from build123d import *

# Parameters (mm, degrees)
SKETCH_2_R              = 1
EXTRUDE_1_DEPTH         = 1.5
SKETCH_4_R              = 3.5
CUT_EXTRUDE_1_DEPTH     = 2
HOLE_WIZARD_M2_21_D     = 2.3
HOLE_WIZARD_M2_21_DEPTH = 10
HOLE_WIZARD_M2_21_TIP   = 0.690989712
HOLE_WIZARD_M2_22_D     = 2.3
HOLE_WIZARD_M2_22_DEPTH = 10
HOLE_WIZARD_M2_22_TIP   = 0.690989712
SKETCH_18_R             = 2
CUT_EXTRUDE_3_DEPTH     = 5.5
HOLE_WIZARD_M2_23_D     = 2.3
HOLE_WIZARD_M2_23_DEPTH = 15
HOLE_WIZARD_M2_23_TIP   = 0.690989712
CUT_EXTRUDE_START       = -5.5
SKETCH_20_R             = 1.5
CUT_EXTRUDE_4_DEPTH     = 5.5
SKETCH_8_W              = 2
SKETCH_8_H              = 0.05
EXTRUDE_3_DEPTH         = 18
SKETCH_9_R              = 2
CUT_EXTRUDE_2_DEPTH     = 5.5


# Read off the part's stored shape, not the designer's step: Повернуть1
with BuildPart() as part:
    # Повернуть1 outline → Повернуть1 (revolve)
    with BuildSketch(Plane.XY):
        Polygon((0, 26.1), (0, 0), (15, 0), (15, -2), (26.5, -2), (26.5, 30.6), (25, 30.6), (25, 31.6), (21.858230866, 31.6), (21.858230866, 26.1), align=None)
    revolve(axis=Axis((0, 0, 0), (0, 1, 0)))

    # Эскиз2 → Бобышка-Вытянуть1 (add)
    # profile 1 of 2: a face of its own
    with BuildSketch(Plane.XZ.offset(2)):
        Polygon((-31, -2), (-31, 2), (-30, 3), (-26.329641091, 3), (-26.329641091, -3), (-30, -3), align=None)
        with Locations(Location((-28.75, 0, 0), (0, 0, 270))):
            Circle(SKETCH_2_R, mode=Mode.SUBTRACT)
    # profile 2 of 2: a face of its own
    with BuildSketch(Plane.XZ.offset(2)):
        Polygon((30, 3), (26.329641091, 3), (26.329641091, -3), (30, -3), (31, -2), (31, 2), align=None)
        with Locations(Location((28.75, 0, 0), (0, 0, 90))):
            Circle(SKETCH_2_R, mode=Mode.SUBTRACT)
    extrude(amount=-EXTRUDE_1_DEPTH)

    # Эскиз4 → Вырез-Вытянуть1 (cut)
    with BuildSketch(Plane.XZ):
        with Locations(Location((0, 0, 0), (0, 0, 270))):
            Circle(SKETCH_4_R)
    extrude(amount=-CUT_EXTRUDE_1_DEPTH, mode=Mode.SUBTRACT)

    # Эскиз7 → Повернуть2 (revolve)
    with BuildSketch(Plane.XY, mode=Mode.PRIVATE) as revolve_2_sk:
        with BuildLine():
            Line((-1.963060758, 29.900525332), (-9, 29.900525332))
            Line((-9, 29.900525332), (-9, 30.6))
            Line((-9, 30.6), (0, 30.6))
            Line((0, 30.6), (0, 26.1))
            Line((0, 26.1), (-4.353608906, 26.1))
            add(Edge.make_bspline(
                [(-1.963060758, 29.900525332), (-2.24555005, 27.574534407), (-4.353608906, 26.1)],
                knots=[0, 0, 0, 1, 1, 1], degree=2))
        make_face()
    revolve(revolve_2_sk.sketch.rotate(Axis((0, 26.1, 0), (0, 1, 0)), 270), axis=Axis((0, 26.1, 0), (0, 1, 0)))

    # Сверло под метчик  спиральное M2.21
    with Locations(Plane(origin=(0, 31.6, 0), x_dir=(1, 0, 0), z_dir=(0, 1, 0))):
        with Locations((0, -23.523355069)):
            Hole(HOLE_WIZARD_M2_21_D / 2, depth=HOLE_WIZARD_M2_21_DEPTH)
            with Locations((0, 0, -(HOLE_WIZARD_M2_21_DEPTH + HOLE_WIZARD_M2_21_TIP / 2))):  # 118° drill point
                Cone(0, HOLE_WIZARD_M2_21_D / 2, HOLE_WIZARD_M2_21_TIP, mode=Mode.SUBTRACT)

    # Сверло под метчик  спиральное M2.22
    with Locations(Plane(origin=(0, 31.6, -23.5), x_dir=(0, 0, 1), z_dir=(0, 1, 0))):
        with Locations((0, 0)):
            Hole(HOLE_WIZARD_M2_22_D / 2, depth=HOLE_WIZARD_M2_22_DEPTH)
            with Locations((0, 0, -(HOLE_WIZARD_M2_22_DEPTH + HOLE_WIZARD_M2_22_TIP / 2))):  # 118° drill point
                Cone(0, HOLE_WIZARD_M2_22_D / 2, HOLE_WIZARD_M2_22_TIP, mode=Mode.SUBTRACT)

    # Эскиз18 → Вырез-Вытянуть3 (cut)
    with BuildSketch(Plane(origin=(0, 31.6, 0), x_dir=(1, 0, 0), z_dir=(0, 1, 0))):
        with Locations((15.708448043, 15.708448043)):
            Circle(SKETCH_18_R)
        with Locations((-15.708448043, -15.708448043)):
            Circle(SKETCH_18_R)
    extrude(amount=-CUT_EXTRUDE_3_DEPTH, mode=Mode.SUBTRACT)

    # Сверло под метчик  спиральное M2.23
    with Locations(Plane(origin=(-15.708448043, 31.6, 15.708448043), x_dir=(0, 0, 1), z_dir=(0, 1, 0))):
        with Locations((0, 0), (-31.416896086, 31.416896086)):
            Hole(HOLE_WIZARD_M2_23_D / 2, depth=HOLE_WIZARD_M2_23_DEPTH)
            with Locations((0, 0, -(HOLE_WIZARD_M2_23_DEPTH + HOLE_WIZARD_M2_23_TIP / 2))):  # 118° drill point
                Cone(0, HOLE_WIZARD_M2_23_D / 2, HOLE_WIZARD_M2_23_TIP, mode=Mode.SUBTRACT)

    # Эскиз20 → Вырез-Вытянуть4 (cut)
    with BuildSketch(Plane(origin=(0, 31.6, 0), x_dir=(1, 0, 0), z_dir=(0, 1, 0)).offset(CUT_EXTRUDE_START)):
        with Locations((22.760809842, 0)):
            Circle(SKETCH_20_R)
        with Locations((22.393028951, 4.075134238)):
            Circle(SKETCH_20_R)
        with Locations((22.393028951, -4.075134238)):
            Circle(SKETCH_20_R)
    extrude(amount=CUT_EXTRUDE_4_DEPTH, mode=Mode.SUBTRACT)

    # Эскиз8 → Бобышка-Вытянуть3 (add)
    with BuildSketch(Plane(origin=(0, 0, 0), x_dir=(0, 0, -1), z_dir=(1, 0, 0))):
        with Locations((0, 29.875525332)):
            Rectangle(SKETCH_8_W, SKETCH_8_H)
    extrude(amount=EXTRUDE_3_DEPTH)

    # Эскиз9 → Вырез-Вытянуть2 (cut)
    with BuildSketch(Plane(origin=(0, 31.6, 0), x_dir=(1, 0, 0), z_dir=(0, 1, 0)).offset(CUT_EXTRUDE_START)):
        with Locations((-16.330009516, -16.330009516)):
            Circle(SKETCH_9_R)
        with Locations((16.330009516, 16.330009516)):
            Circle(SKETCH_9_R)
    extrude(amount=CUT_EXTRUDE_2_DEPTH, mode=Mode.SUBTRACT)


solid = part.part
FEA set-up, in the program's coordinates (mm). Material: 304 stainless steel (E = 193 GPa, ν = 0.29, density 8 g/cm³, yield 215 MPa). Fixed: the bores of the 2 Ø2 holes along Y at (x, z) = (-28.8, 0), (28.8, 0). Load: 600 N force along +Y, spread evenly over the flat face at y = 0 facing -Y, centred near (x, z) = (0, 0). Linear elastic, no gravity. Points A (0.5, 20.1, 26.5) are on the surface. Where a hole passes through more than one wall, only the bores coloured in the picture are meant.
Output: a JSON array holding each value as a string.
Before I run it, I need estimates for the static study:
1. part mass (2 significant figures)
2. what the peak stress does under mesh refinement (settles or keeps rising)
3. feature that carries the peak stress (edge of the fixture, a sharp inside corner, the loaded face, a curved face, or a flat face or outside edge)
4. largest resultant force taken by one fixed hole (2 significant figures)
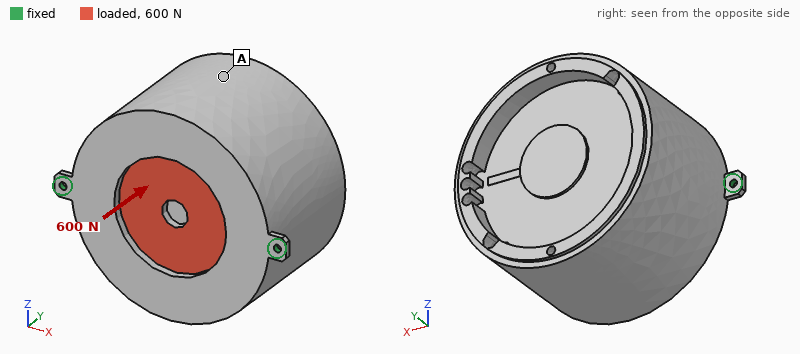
["510 g", "keeps rising", "edge of the fixture", "340 N"]
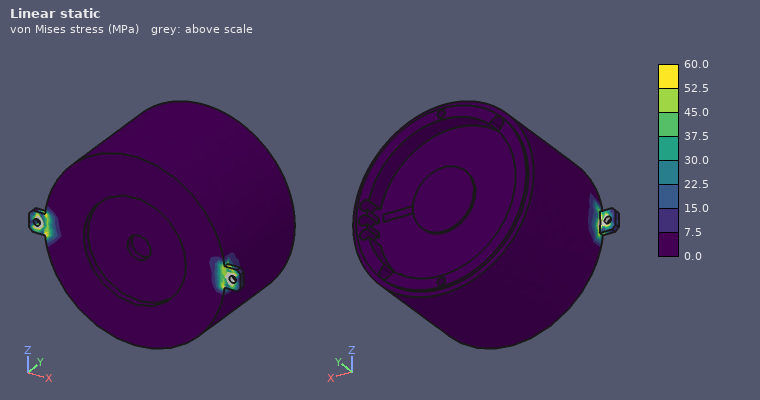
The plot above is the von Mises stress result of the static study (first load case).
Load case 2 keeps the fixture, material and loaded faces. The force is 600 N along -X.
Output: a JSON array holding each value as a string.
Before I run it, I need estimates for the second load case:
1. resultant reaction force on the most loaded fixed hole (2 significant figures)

["300 N"]
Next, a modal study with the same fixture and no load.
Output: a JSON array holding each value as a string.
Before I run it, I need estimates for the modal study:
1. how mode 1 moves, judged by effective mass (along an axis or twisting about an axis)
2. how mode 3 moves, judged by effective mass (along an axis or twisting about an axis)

["along Z", "along Y"]
